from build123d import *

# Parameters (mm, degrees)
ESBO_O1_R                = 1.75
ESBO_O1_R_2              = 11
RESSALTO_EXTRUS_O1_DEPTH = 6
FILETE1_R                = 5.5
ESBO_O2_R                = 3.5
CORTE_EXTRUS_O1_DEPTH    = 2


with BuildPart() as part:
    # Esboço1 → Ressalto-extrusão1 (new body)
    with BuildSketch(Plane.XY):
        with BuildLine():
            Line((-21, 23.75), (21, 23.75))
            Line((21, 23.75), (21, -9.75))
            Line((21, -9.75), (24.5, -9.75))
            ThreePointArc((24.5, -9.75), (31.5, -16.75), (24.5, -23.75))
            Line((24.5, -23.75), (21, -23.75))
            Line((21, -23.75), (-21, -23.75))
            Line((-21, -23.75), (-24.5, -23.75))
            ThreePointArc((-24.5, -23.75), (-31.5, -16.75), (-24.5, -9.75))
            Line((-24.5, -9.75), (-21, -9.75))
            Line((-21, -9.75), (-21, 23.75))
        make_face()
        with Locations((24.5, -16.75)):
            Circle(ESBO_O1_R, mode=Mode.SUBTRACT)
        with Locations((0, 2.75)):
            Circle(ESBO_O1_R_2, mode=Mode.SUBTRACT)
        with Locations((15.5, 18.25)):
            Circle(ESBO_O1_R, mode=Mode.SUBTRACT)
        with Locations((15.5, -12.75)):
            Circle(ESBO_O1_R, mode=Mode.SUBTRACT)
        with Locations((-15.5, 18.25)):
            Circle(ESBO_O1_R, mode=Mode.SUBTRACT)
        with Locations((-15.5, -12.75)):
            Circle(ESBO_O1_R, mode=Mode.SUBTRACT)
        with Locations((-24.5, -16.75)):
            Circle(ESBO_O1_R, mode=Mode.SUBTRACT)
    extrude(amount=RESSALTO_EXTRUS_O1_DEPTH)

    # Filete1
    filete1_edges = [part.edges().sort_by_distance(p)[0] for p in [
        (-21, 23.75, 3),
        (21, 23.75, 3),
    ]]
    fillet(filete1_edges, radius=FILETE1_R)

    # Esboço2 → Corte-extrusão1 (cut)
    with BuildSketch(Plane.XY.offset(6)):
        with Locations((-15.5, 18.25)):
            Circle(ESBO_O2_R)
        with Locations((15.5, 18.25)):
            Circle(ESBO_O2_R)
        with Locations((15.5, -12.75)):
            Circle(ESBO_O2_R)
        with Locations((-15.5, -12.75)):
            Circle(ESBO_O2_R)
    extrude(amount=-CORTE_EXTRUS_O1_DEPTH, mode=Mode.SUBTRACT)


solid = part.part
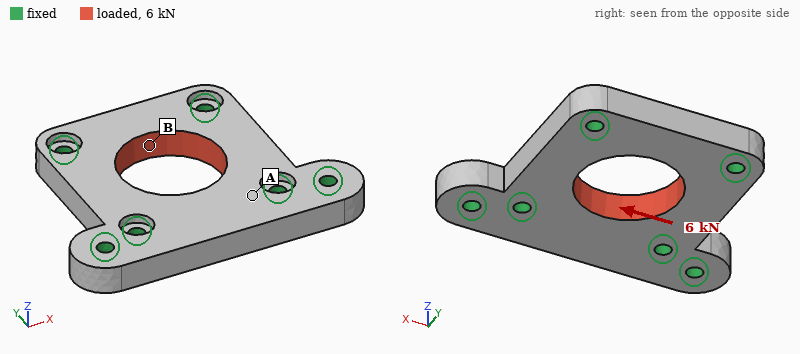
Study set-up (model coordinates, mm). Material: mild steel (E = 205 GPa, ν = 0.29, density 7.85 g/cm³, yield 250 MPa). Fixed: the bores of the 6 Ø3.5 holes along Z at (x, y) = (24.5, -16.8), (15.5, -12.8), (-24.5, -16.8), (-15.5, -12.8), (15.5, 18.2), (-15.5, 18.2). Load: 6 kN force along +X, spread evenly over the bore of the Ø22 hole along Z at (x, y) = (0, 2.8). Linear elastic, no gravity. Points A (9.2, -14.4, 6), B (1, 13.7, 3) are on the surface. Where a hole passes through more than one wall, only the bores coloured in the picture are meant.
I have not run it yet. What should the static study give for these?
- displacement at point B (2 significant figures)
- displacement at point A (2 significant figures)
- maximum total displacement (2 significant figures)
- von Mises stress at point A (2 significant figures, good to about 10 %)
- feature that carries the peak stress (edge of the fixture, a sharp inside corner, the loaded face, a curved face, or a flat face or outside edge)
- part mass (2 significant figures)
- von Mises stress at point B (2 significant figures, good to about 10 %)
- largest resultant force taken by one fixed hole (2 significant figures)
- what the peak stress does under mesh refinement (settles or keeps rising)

1.6 µm
0.61 µm
3.3 µm
12 MPa
edge of the fixture
83 g
27 MPa
1.5 kN
keeps rising
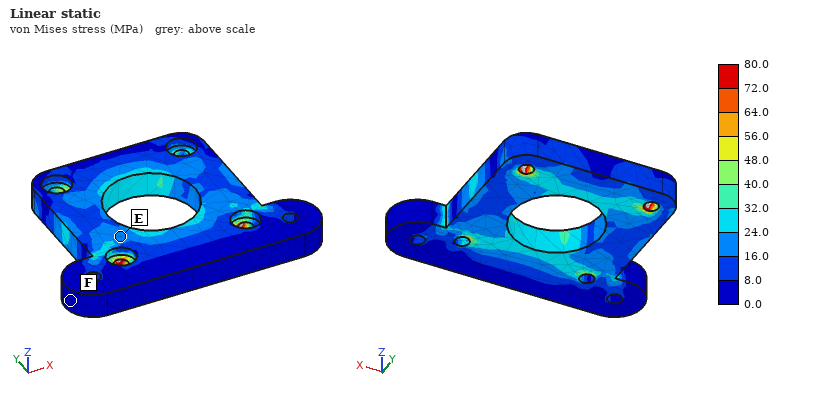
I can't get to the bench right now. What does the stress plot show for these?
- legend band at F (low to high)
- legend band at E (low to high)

0.0 to 8.0 MPa
16.0 to 24.0 MPa
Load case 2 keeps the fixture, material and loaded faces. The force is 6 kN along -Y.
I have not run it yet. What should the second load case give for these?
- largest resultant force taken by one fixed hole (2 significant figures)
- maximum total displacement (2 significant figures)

1.5 kN
3.7 µm
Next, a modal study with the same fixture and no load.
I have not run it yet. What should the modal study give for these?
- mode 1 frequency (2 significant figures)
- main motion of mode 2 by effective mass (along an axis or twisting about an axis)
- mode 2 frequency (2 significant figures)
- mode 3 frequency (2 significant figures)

20 kHz
along Z
22 kHz
25 kHz
